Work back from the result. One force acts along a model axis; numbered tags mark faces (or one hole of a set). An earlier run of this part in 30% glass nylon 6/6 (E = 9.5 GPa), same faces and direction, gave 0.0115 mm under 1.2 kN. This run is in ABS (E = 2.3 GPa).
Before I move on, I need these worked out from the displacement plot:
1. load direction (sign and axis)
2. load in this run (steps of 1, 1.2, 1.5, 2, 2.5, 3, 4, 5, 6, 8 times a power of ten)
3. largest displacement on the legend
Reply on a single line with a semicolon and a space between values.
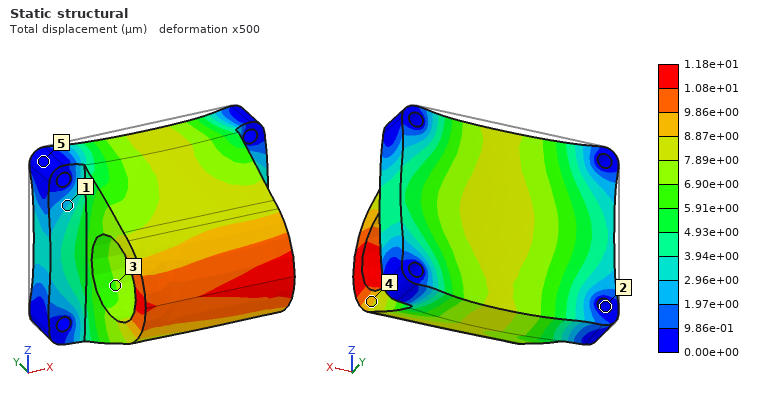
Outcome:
-Y; 300 N; 1.18e+01 µm
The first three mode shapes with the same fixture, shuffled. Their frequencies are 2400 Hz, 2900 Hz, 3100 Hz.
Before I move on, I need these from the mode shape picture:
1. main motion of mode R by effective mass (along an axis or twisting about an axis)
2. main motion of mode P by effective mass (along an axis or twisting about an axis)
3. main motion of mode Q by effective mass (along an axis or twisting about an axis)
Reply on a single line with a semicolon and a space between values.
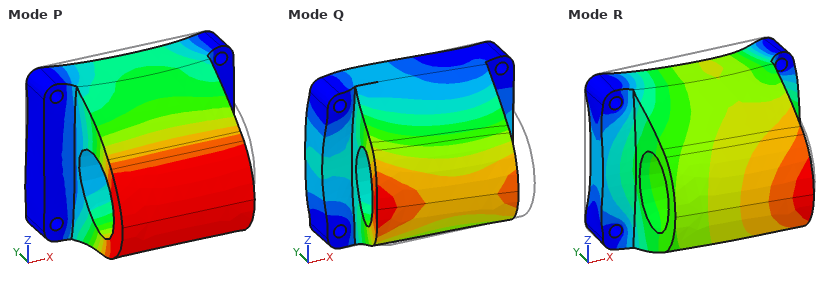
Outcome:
along Y; along Z; along X
